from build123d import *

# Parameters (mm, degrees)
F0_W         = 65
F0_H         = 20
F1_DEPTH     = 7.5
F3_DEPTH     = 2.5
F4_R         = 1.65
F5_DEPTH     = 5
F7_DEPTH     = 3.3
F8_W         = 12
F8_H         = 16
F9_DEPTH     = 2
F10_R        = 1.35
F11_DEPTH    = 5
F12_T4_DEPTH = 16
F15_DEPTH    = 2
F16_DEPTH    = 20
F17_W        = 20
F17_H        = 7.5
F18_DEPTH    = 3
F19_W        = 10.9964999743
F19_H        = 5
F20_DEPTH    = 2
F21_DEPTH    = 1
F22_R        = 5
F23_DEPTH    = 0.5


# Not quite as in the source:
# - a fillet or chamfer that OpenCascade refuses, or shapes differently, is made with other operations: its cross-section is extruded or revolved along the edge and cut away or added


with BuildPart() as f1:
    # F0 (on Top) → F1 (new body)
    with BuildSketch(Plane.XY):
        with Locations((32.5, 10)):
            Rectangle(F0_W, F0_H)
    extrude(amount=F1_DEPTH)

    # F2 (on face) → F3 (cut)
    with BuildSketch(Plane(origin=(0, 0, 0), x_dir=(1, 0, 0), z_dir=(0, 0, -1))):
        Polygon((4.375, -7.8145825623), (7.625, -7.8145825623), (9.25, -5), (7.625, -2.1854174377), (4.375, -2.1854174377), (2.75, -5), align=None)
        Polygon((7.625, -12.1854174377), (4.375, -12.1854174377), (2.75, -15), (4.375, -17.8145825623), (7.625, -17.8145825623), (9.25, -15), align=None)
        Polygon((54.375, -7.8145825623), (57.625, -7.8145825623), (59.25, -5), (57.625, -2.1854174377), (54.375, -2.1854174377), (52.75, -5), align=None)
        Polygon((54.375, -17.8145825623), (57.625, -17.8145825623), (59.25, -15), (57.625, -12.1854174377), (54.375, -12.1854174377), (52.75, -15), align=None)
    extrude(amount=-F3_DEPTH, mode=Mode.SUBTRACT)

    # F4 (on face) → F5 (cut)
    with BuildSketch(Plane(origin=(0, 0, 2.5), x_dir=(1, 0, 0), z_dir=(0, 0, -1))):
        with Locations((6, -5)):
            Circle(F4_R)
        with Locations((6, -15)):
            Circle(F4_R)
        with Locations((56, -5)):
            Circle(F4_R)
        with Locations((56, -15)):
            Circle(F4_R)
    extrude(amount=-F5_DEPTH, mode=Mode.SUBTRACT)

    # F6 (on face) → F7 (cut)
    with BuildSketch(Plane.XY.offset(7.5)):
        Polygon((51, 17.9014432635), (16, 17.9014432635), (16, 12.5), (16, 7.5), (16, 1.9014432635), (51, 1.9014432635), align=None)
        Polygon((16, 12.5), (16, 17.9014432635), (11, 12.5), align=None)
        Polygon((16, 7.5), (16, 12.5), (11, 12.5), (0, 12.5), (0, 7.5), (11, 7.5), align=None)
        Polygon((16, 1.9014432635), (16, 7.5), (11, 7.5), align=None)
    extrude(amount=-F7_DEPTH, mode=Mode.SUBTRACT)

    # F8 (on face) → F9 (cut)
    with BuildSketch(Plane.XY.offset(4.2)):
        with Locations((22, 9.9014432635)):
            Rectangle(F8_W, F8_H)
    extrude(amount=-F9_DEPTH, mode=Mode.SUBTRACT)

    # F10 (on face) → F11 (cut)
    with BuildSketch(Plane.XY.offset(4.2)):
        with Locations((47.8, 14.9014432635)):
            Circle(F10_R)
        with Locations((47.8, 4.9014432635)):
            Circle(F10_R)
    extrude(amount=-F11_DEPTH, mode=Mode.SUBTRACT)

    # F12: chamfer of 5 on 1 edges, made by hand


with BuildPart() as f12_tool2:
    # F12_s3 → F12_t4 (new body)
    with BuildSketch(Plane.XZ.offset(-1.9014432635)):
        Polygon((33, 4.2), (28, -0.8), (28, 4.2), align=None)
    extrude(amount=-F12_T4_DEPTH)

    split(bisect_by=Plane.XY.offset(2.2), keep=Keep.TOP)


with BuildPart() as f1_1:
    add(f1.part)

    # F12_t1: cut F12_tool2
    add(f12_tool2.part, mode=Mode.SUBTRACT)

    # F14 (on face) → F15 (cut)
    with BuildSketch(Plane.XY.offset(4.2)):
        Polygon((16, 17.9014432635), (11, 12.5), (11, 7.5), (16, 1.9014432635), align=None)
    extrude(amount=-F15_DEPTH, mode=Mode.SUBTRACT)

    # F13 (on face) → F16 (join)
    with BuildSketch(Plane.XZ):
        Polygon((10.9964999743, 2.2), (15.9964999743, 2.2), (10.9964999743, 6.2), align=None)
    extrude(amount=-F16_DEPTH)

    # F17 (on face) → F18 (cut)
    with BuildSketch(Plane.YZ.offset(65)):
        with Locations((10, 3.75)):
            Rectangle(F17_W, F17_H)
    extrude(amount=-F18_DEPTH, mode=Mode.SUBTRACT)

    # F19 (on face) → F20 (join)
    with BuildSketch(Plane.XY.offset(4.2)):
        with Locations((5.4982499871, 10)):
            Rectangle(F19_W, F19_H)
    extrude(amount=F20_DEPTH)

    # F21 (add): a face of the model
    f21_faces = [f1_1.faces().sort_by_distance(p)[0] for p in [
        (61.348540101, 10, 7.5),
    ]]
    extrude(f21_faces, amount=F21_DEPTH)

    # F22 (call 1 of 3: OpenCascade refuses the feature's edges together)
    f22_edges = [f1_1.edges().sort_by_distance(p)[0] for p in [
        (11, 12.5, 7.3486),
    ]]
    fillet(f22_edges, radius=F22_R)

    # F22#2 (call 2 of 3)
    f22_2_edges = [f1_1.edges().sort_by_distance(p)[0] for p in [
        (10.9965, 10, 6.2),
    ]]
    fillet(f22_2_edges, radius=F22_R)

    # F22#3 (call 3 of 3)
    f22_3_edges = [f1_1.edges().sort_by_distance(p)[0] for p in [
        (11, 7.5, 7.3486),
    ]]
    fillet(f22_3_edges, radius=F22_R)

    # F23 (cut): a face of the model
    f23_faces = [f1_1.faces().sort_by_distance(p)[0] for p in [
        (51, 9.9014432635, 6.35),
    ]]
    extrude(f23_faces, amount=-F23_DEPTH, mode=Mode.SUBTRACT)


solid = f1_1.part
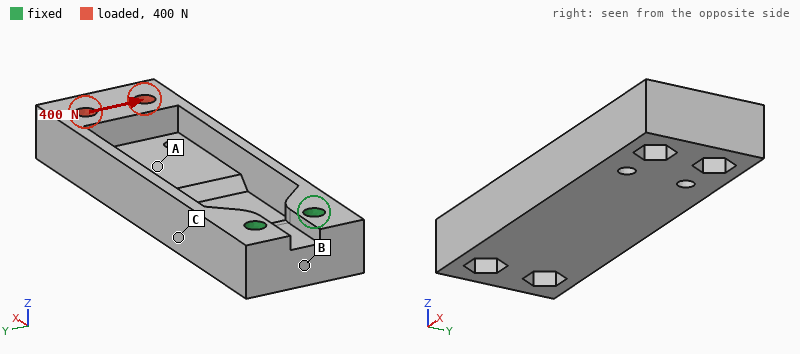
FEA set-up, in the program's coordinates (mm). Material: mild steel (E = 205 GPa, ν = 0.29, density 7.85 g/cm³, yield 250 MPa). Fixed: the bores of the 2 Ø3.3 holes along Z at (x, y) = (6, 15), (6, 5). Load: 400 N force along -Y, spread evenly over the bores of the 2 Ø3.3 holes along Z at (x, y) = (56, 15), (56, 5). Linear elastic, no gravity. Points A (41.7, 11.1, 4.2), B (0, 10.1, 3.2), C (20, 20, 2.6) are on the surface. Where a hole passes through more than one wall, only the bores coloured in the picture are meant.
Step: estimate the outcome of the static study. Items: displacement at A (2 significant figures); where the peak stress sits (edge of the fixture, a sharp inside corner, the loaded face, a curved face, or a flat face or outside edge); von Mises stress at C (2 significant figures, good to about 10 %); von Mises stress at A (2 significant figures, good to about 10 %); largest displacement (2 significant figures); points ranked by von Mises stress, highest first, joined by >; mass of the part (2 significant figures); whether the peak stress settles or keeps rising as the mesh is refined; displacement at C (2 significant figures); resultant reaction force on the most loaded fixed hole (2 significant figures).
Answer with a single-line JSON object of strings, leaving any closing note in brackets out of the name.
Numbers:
{"displacement at A": "30 µm", "where the peak stress sits": "edge of the fixture", "von Mises stress at C": "61 MPa", "von Mises stress at A": "39 MPa", "largest displacement": "66 µm", "points ranked by von Mises stress, highest first, joined by >": "C > A > B", "mass of the part": "52 g", "whether the peak stress settles or keeps rising as the mesh is refined": "keeps rising", "displacement at C": "10 µm", "resultant reaction force on the most loaded fixed hole": "1.5 kN"}
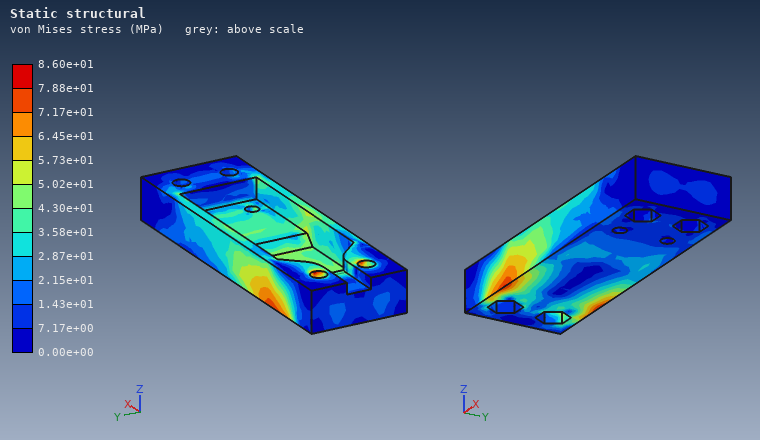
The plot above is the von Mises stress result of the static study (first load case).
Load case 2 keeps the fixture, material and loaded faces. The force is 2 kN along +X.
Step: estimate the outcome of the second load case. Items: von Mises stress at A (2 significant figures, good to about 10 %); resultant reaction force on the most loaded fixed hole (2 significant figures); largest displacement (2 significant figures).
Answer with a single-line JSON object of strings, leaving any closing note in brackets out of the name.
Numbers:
{"von Mises stress at A": "35 MPa", "resultant reaction force on the most loaded fixed hole": "1.0 kN", "largest displacement": "95 µm"}
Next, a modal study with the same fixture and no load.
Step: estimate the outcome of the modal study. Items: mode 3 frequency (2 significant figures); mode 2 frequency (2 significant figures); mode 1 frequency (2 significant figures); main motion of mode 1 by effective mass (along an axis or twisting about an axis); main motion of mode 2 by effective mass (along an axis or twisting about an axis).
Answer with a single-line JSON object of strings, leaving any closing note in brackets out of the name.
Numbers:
{"mode 3 frequency": "6100 Hz", "mode 2 frequency": "3200 Hz", "mode 1 frequency": "1600 Hz", "main motion of mode 1 by effective mass": "along Z", "main motion of mode 2 by effective mass": "along Y"}
